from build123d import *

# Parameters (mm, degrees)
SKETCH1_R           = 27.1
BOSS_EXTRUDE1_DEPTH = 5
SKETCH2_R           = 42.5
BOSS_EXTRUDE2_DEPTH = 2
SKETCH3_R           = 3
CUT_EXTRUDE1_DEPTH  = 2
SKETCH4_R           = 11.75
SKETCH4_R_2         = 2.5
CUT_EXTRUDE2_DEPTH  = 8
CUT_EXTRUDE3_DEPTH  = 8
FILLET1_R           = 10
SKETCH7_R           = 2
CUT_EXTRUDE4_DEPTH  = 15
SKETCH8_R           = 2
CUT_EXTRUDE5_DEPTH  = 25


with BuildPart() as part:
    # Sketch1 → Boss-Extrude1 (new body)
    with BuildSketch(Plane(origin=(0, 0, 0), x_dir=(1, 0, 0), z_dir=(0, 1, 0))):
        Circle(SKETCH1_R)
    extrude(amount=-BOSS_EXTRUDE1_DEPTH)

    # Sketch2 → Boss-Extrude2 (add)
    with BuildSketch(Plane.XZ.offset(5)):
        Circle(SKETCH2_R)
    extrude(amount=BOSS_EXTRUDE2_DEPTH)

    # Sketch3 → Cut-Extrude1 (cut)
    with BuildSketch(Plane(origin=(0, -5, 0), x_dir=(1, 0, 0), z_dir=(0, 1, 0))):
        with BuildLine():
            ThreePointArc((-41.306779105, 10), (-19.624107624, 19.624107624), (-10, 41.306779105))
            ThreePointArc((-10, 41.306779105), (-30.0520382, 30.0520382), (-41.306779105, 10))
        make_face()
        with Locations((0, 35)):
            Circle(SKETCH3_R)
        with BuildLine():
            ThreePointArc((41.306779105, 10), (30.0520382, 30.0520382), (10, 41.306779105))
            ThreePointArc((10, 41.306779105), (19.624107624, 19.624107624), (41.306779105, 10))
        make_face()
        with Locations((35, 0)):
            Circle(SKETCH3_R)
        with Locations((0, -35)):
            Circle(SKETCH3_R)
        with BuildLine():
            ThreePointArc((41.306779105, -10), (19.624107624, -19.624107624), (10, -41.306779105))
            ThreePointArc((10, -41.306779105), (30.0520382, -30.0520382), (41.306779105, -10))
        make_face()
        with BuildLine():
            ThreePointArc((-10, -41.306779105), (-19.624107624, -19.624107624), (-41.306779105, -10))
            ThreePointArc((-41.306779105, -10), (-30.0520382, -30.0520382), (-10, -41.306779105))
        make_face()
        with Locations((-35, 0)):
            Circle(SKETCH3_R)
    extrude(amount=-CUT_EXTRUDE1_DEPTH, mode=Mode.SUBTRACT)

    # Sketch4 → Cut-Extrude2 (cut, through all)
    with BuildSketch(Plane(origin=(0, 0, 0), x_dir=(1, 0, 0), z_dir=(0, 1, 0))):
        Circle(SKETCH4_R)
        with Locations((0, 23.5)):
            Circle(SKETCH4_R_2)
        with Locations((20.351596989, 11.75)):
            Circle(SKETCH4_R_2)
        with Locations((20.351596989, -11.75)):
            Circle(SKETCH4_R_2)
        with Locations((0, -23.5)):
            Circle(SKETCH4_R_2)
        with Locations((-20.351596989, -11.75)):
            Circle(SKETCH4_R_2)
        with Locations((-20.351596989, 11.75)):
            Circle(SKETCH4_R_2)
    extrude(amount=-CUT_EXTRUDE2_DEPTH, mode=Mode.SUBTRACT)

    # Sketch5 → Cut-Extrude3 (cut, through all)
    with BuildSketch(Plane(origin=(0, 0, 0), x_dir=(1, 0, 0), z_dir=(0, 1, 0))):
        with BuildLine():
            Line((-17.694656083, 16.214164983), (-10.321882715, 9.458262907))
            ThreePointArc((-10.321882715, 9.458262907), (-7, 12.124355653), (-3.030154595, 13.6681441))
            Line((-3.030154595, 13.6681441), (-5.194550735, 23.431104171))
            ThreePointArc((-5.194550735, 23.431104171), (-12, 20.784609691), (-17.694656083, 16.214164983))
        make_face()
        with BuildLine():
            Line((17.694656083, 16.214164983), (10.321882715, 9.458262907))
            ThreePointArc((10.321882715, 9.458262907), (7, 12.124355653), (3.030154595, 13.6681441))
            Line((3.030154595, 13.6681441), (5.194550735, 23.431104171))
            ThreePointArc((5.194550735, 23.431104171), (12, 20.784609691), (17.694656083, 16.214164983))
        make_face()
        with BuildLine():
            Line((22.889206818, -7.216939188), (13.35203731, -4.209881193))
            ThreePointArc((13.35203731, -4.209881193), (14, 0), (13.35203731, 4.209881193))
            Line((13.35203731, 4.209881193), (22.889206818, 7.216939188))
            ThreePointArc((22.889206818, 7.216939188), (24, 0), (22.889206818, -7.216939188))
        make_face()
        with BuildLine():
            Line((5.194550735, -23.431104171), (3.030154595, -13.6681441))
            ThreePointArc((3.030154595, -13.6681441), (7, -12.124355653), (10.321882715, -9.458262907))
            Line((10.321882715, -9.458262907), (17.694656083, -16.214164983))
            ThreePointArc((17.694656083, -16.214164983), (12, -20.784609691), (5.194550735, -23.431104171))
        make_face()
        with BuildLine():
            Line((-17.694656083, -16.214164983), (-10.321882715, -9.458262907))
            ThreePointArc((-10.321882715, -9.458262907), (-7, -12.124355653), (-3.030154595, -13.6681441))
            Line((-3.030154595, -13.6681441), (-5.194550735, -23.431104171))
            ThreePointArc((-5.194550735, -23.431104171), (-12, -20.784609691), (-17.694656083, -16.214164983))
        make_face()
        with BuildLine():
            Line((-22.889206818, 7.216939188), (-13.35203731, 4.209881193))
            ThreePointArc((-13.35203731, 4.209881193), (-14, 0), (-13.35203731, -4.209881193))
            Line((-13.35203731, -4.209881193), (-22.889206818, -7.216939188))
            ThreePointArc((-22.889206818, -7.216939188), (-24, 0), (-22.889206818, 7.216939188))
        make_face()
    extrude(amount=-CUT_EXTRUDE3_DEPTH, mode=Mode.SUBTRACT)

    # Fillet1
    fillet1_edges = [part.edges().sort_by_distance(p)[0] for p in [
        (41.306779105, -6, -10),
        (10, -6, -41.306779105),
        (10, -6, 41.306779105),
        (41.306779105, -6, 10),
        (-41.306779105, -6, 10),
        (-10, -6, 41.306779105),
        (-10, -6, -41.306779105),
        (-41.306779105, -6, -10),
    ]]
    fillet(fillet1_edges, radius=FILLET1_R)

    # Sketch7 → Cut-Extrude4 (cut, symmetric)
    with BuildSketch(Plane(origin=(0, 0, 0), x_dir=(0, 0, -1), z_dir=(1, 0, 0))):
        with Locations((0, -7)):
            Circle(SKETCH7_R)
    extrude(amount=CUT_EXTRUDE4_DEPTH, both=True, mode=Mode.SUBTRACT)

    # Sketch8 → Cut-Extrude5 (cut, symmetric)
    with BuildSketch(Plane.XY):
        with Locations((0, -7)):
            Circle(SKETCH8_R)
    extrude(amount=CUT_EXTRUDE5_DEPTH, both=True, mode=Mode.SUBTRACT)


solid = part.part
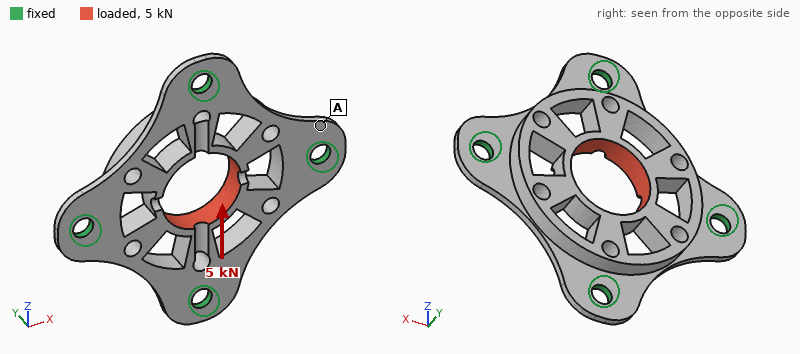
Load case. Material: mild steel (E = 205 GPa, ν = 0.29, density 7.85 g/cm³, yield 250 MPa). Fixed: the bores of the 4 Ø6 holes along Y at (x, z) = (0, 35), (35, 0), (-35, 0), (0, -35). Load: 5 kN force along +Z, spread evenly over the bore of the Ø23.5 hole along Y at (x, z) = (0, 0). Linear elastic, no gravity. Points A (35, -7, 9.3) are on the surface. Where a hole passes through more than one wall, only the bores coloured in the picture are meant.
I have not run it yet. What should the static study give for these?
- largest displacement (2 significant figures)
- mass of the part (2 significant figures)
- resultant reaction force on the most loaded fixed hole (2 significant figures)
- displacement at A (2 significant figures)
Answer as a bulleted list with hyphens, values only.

- 18 µm
- 79 g
- 1.6 kN
- 3.4 µm
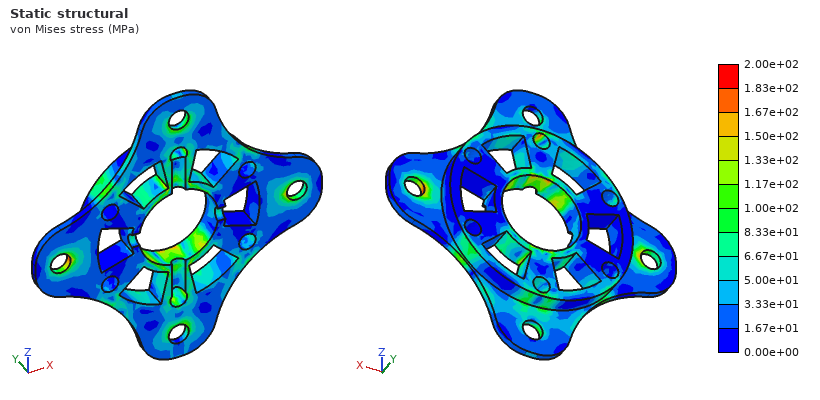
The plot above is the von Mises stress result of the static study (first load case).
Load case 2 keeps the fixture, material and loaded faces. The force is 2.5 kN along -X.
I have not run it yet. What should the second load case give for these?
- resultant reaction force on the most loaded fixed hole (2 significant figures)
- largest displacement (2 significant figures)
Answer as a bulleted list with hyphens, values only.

- 890 N
- 6.7 µm
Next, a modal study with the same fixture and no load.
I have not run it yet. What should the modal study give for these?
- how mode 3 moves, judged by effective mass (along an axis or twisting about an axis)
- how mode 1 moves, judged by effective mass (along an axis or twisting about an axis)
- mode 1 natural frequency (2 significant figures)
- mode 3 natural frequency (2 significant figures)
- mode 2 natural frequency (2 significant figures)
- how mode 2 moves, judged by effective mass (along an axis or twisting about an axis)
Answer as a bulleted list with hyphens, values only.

- twisting about Z
- along Y
- 6100 Hz
- 8700 Hz
- 8300 Hz
- twisting about X
